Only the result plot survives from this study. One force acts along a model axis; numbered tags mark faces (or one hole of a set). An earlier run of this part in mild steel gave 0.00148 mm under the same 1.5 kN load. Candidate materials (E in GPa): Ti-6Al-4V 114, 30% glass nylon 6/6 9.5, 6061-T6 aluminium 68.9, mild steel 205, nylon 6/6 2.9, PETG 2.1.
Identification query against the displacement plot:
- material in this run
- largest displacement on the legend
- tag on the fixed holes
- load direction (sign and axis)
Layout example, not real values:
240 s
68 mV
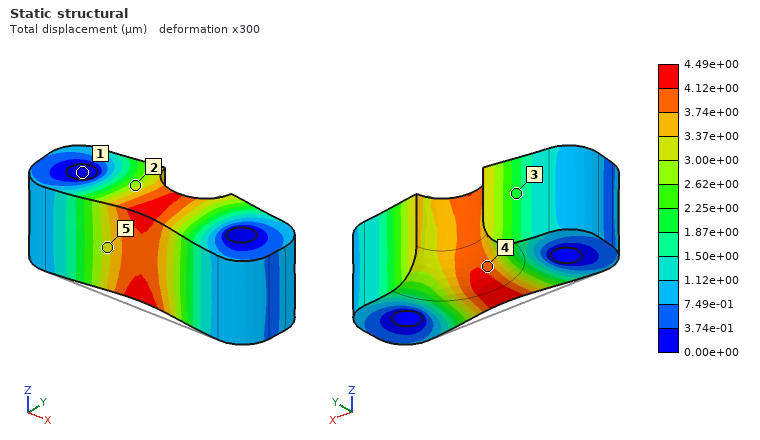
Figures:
6061-T6 aluminium
4.49e+00 µm
1
+Y
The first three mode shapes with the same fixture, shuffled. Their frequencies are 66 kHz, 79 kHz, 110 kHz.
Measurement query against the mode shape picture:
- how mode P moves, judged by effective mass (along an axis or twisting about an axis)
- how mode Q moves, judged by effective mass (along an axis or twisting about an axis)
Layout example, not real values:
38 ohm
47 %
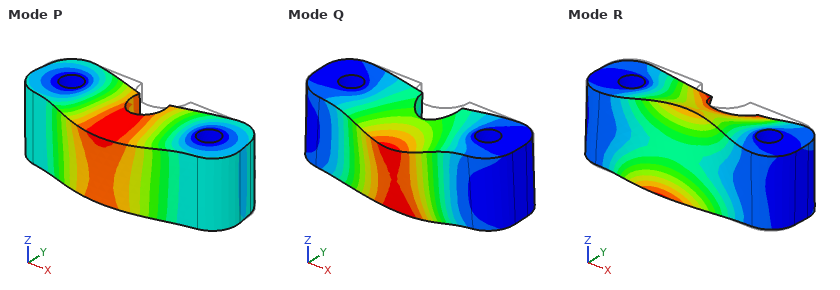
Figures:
along Y
along Z
